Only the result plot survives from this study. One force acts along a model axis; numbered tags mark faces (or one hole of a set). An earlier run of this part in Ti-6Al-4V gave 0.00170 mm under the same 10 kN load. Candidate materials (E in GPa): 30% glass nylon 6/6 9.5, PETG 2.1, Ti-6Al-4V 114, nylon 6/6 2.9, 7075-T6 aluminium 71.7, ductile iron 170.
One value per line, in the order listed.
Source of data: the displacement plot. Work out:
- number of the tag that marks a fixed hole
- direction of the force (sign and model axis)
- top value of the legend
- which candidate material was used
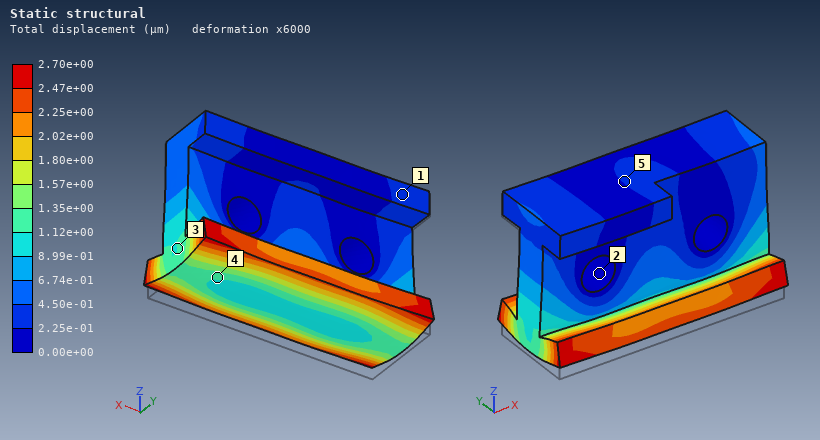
2
+Z
2.70e+00 µm
7075-T6 aluminium
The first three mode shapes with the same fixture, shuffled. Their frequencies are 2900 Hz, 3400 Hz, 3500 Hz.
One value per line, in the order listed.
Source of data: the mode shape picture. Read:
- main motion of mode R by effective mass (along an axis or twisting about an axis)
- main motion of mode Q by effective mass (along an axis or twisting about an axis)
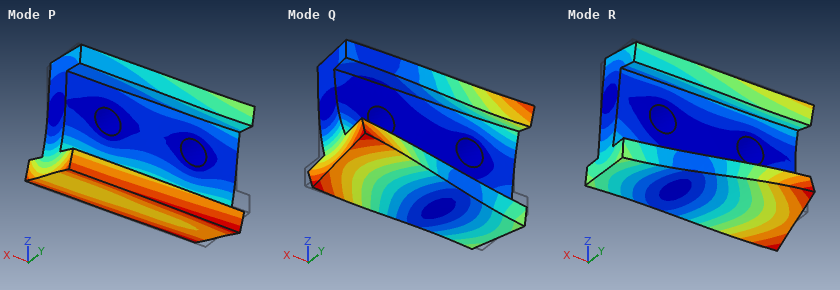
along Y
along Y
